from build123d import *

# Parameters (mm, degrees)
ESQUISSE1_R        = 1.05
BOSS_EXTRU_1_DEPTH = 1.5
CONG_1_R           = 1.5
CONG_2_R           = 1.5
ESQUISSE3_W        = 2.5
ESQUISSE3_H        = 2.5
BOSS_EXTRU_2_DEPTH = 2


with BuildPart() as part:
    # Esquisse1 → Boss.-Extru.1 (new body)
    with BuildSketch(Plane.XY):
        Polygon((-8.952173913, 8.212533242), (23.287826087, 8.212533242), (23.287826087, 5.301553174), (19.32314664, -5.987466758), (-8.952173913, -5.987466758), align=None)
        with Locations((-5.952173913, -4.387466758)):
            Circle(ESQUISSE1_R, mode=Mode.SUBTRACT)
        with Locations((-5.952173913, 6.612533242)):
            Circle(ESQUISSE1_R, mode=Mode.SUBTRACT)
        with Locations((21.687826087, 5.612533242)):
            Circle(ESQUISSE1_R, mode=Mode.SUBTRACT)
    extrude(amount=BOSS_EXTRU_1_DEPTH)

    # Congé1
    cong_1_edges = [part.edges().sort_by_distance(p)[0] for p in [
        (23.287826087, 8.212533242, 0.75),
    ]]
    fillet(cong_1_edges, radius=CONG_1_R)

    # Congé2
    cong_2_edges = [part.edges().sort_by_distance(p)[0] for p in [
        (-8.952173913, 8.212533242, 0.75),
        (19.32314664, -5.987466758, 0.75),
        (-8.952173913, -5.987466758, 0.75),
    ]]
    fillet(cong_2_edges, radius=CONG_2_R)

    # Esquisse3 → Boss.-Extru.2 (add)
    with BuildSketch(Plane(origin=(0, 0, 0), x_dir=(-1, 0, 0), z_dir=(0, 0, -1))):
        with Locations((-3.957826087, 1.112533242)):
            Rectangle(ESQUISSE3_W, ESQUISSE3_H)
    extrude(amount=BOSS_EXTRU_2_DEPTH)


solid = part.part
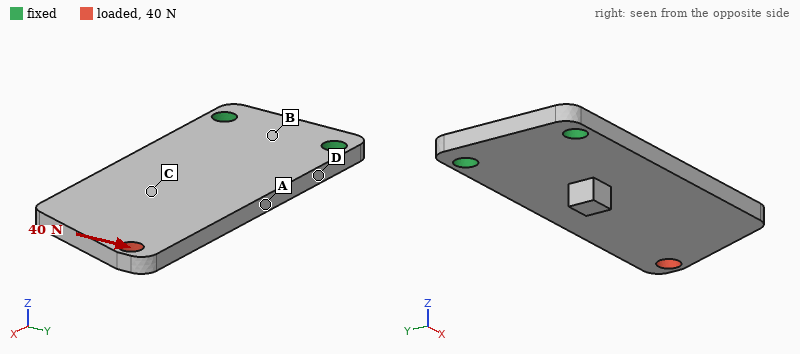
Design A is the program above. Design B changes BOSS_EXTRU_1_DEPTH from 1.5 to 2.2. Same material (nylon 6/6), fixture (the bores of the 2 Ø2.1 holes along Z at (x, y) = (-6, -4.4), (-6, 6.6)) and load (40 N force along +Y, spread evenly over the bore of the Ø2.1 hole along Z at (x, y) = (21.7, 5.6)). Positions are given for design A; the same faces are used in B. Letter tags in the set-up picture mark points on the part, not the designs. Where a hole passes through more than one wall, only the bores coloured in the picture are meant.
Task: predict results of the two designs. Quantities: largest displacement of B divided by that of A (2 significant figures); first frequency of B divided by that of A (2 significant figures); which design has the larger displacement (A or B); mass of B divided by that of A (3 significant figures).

0.68
1.4
A
1.46
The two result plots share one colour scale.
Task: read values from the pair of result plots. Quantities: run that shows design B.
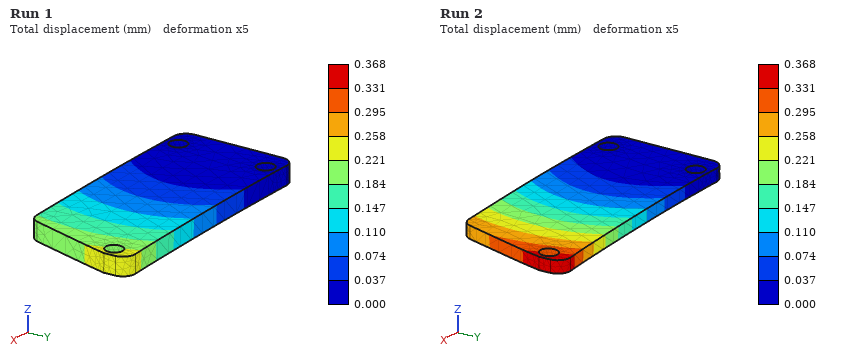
Run 1
